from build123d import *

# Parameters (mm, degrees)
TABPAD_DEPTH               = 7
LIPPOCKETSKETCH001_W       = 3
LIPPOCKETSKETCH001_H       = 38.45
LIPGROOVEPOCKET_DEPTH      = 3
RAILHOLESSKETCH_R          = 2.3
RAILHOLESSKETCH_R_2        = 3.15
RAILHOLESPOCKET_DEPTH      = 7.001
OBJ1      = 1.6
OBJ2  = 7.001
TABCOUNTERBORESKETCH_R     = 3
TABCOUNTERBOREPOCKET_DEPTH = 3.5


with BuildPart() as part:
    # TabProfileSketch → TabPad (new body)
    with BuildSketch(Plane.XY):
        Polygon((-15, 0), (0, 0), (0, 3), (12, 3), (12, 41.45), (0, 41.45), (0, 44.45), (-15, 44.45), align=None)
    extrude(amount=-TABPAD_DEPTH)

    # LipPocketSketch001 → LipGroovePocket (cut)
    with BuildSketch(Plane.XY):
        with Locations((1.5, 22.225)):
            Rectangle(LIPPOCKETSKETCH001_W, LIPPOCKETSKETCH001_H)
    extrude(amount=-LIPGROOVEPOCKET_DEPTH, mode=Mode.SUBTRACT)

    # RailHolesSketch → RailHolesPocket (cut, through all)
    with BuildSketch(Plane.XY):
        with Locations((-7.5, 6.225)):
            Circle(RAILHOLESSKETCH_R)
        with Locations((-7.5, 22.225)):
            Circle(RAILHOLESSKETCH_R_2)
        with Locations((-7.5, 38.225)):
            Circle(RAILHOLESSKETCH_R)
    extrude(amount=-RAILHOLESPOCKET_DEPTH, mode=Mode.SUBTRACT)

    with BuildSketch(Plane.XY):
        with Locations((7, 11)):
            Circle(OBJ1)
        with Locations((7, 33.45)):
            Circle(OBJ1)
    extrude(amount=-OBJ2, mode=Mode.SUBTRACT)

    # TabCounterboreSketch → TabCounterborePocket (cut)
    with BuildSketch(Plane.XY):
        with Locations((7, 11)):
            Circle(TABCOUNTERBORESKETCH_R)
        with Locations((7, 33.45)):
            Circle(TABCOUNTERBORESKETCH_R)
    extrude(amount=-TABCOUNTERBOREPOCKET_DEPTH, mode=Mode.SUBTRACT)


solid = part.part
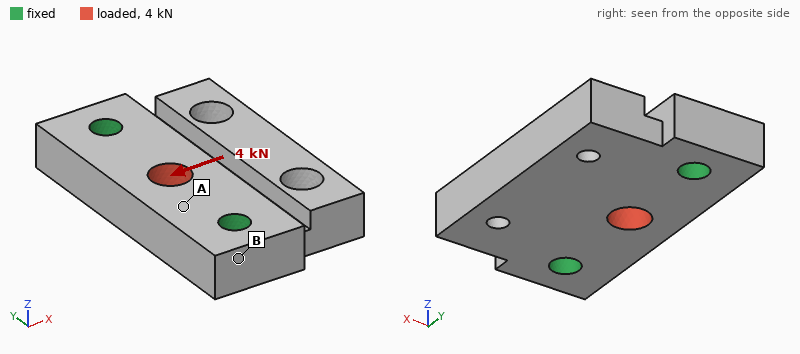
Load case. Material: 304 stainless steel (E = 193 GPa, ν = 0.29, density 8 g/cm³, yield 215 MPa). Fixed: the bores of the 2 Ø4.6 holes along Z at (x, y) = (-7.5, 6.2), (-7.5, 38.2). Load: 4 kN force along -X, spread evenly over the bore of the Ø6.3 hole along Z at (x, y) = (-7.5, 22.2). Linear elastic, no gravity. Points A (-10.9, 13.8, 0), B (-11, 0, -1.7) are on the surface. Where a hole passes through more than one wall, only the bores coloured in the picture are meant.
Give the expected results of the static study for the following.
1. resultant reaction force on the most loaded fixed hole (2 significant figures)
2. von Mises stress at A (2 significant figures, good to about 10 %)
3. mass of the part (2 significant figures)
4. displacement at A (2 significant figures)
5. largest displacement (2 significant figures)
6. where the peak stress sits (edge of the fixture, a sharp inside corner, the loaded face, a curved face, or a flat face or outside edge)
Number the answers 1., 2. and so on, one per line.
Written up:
1. 2.0 kN
2. 27 MPa
3. 55 g
4. 2.5 µm
5. 5.5 µm
6. edge of the fixture
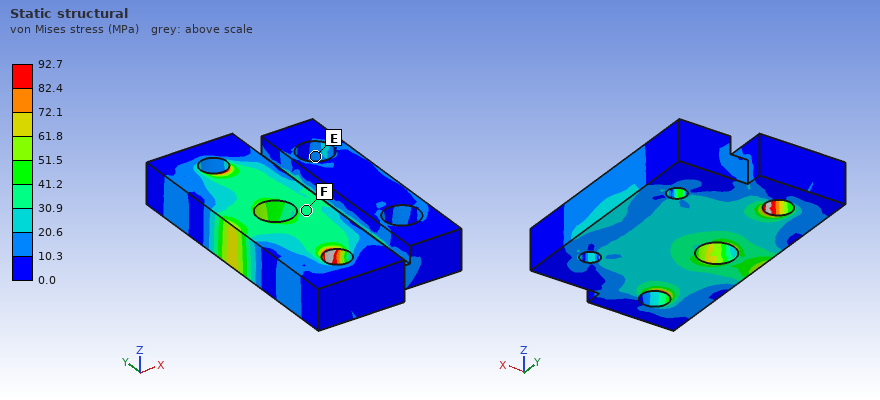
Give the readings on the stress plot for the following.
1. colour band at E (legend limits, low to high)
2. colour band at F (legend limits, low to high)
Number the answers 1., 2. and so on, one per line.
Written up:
1. 10.3 to 20.6 MPa
2. 30.9 to 41.2 MPa
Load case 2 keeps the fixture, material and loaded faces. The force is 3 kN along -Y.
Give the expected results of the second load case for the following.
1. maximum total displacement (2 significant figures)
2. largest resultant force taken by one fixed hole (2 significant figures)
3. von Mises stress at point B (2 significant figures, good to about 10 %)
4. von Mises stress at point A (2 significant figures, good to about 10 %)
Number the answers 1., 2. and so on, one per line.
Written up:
1. 1.4 µm
2. 1.5 kN
3. 4.3 MPa
4. 17 MPa
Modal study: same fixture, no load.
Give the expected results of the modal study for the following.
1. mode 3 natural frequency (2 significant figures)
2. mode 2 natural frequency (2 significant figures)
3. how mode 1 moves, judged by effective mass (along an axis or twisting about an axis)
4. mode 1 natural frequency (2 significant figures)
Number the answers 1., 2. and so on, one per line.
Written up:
1. 26 kHz
2. 17 kHz
3. along Z
4. 9500 Hz
